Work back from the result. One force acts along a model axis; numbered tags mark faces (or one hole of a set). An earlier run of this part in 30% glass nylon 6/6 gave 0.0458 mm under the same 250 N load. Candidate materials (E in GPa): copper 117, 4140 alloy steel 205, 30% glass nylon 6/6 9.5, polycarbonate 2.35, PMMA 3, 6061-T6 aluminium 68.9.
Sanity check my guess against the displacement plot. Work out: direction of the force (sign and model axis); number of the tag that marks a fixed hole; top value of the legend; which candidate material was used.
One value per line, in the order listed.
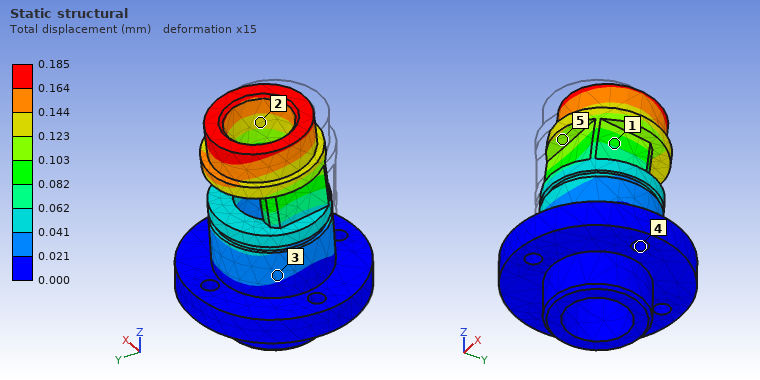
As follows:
+Y
4
0.185 mm
polycarbonate
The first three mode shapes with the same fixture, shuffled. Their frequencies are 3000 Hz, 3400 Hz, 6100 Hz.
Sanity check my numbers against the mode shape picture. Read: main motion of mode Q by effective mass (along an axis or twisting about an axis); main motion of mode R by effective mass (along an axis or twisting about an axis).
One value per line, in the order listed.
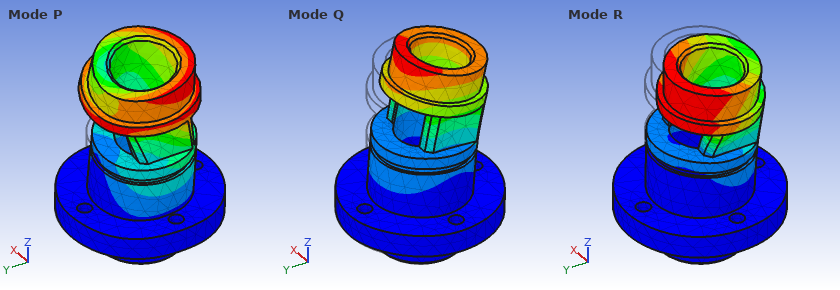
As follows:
along Y
along X
